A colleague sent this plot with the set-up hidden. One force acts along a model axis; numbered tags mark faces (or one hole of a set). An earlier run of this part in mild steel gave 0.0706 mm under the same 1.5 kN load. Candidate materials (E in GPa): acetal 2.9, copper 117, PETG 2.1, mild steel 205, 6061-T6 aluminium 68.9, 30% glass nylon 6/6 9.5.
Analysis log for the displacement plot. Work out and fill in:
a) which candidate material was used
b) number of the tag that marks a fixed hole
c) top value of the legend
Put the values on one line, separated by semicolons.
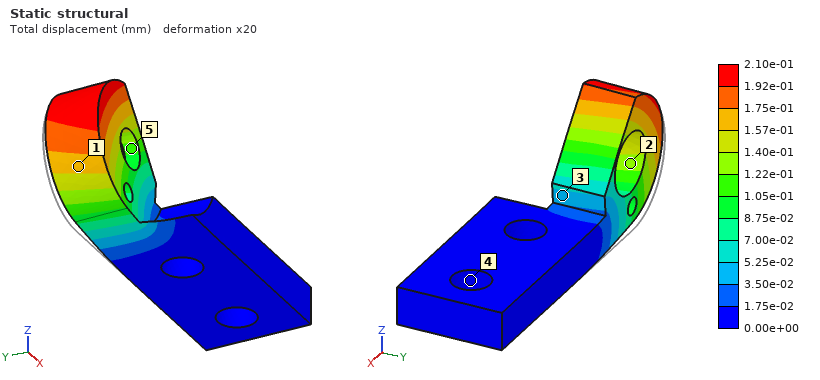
6061-T6 aluminium; 4; 2.10e-01 mm
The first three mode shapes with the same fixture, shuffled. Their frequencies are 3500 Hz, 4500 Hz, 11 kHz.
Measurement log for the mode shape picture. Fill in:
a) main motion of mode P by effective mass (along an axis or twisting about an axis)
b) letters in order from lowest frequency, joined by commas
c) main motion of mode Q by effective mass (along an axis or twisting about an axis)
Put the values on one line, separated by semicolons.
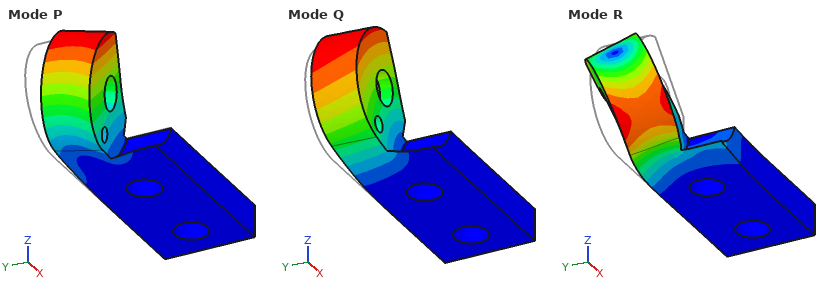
along Y; Q, P, R; along Z
